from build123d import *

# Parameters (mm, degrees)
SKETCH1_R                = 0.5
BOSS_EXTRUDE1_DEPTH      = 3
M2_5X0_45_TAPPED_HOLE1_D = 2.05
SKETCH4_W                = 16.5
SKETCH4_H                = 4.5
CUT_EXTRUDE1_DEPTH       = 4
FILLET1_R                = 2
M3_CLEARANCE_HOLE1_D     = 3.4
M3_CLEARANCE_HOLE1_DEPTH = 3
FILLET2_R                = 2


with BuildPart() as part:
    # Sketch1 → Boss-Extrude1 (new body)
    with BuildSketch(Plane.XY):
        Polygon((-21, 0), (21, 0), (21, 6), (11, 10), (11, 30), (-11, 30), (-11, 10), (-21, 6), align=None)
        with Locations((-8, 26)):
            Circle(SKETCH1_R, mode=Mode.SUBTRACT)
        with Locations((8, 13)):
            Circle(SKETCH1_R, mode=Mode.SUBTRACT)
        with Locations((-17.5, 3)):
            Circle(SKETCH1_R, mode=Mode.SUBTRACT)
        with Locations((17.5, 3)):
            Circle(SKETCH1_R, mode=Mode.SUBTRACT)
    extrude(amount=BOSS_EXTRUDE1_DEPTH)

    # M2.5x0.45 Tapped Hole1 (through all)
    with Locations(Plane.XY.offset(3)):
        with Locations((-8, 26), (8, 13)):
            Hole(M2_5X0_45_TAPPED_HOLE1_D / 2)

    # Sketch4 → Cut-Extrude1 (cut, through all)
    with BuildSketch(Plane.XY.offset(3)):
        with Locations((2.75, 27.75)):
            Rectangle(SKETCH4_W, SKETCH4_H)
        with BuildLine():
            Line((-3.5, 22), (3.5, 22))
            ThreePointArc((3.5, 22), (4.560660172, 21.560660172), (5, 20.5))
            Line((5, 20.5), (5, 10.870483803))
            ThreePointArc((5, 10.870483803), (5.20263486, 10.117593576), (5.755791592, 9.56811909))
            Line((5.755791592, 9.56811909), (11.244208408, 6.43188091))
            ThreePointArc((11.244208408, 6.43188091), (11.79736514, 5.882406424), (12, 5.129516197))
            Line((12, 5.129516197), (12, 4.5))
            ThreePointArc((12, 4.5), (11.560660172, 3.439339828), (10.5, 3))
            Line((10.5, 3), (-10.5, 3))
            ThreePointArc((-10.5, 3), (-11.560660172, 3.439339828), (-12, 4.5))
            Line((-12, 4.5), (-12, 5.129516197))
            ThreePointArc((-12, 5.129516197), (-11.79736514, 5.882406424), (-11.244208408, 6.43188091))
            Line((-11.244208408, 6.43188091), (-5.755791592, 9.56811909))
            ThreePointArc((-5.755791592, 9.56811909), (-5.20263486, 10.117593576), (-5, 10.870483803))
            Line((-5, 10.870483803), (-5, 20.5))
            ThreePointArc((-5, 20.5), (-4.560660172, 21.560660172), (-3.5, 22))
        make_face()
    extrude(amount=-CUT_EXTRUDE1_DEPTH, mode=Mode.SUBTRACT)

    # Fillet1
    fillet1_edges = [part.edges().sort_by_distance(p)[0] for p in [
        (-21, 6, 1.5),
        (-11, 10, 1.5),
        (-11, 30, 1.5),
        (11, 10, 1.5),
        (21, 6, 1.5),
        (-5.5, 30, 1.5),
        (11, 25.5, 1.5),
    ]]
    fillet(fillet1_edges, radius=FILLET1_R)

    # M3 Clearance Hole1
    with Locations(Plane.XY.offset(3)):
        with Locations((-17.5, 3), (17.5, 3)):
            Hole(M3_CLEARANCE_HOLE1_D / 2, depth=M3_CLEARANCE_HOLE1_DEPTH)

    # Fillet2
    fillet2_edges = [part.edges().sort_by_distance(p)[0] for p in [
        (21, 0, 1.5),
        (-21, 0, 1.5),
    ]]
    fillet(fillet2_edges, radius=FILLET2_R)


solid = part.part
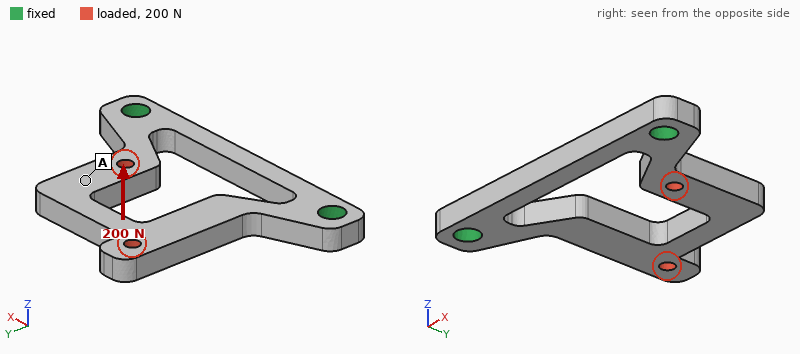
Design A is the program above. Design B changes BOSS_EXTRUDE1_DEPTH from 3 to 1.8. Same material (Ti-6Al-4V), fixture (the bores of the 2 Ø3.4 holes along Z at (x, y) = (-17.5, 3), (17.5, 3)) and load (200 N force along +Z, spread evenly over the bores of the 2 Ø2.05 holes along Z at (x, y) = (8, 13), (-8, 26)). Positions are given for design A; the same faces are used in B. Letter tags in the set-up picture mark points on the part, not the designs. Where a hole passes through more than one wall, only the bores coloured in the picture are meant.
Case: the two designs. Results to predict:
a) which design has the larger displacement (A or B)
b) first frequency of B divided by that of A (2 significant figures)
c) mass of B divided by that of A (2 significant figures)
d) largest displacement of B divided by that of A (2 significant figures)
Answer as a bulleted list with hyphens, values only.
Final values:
- B
- 0.64
- 0.60
- 4.0
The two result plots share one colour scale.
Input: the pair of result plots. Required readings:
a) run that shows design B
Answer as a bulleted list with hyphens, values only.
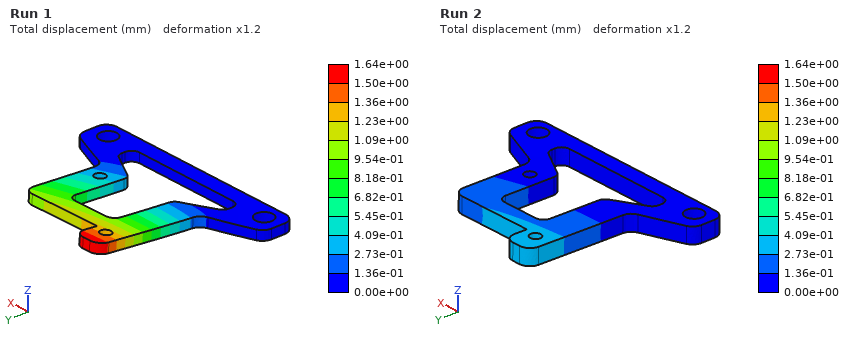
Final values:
- Run 1
